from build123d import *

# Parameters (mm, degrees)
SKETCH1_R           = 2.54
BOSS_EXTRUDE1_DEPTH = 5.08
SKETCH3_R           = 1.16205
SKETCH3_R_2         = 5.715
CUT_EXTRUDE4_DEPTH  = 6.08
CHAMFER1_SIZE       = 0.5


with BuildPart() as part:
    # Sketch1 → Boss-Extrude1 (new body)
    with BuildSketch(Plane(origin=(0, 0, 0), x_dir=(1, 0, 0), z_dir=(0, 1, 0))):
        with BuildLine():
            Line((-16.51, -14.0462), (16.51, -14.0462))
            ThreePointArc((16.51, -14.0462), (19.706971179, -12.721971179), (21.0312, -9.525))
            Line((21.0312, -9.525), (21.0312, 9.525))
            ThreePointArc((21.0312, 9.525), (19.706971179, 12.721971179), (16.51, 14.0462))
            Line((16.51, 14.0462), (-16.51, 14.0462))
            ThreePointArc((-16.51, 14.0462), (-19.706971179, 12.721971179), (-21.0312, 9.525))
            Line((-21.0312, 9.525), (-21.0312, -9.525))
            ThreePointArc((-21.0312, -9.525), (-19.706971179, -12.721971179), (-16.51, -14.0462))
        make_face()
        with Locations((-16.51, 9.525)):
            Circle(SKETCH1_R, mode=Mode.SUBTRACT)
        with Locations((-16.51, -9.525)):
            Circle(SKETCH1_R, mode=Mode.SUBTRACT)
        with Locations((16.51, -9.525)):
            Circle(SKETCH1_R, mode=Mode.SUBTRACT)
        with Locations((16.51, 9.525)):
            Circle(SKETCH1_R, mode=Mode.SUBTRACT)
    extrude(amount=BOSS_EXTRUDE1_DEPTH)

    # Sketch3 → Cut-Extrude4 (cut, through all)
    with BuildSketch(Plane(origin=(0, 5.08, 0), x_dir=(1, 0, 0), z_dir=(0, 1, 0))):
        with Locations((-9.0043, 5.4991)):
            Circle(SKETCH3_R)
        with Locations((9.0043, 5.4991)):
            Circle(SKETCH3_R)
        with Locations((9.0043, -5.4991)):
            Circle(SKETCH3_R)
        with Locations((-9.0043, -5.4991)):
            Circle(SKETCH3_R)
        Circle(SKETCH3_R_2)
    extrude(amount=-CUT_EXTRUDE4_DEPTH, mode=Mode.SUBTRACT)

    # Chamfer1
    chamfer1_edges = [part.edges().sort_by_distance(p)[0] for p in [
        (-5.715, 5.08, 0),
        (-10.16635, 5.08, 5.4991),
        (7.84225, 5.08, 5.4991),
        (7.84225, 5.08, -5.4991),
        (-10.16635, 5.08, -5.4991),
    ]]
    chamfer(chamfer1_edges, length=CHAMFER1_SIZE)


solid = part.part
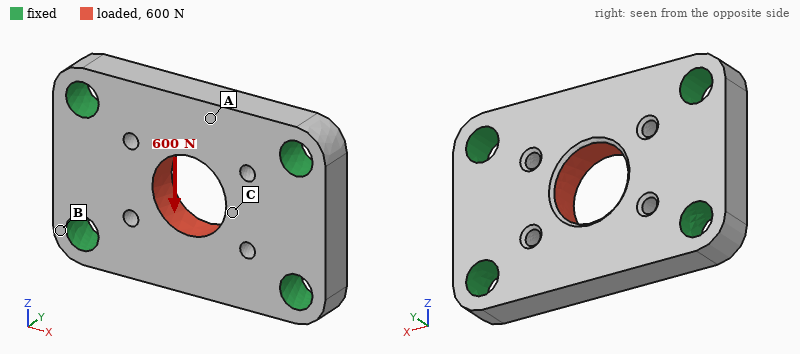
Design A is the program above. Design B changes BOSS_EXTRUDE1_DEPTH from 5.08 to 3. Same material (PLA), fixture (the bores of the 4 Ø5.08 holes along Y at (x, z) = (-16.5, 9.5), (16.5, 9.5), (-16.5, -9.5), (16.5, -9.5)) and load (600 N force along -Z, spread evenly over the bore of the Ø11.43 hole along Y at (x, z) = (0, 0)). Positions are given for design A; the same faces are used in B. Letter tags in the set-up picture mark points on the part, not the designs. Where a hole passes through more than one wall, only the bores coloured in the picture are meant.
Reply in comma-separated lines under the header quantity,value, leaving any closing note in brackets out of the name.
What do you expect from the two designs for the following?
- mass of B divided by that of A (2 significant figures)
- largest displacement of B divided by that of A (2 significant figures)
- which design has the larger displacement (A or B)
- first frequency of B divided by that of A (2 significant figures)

quantity,value
mass of B divided by that of A,0.59
largest displacement of B divided by that of A,1.7
which design has the larger displacement,B
first frequency of B divided by that of A,0.68
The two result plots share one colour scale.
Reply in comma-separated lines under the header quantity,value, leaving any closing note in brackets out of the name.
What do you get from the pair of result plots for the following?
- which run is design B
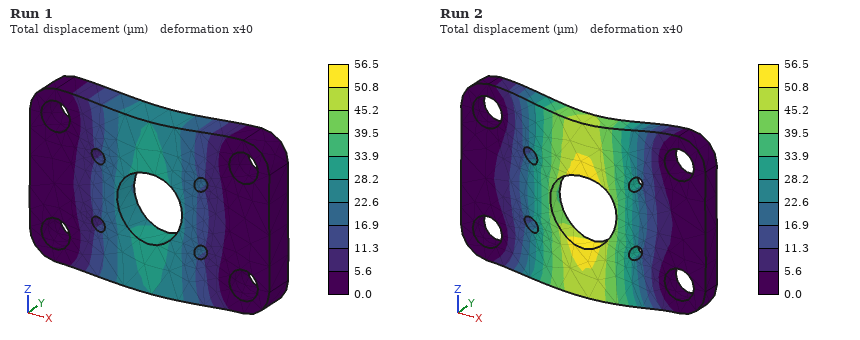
quantity,value
which run is design B,Run 2
